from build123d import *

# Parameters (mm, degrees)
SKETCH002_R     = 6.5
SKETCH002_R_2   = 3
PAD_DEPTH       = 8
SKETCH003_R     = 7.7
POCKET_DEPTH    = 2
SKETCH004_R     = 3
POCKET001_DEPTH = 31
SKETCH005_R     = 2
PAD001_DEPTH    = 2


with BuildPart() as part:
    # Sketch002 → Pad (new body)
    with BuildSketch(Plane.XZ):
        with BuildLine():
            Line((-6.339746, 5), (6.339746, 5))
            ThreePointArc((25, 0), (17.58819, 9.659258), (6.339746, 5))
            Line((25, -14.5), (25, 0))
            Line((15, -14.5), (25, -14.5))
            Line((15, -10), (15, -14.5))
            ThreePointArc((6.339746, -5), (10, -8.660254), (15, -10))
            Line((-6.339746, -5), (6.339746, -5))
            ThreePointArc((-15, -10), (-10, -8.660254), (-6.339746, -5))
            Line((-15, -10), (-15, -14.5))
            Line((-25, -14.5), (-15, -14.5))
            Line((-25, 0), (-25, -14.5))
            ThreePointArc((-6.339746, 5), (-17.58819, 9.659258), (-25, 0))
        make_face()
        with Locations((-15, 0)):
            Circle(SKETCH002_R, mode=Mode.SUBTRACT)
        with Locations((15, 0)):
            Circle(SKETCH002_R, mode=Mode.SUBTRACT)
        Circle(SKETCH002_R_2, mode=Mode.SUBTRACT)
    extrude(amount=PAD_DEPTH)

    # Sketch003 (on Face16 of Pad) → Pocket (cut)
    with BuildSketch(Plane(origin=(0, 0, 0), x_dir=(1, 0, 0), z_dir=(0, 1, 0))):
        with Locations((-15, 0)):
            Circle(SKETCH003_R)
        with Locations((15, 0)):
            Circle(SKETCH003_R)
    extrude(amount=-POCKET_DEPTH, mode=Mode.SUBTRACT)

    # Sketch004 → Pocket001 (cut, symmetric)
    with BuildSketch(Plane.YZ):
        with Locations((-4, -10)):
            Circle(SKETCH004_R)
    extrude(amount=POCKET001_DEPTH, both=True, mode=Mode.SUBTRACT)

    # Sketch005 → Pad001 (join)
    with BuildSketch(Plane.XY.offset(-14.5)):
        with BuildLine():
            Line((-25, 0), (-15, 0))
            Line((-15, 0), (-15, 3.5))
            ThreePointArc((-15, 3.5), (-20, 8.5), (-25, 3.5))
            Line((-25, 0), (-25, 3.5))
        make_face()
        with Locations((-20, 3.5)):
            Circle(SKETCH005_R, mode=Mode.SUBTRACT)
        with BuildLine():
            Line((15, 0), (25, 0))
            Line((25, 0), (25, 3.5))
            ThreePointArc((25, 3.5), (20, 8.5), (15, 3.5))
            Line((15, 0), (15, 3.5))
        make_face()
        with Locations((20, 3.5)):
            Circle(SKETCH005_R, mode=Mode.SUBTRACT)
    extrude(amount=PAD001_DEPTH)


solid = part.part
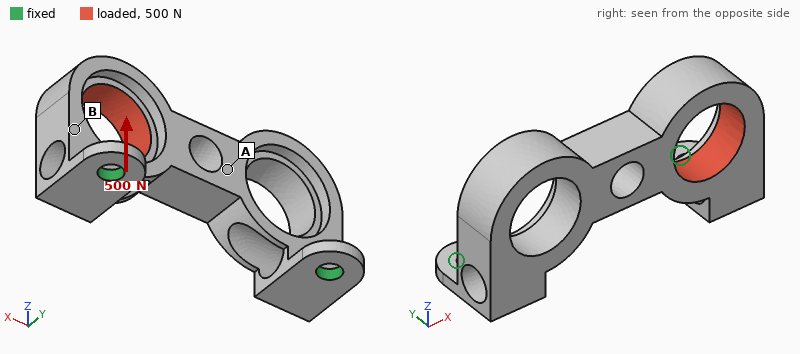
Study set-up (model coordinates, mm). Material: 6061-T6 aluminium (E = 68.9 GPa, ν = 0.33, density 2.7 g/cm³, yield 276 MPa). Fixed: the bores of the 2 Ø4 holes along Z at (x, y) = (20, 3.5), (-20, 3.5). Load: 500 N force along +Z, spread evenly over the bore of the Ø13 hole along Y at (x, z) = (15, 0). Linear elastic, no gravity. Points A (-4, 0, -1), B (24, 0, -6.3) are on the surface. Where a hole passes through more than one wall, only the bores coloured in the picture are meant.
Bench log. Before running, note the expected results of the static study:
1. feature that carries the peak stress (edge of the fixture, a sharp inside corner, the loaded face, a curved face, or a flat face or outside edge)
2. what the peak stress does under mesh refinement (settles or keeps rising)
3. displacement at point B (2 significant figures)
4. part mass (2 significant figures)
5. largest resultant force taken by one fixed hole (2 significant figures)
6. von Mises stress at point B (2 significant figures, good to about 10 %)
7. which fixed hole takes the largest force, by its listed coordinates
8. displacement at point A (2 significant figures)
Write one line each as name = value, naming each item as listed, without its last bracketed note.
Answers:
feature that carries the peak stress = a sharp inside corner
what the peak stress does under mesh refinement = keeps rising
displacement at point B = 0.099 mm
part mass = 11 g
largest resultant force taken by one fixed hole = 430 N
von Mises stress at point B = 46 MPa
which fixed hole takes the largest force, by its listed coordinates = (20, 3.5)
displacement at point A = 0.15 mm
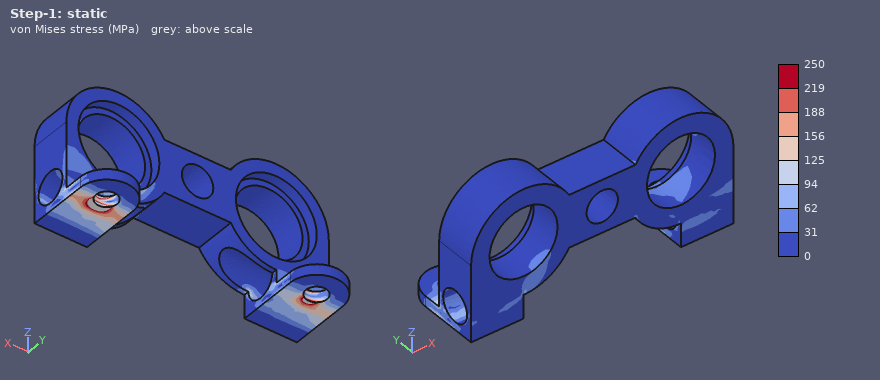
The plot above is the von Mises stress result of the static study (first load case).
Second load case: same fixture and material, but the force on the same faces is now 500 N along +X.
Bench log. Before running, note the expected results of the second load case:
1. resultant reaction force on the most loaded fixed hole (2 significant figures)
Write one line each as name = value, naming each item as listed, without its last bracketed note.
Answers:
resultant reaction force on the most loaded fixed hole = 300 N
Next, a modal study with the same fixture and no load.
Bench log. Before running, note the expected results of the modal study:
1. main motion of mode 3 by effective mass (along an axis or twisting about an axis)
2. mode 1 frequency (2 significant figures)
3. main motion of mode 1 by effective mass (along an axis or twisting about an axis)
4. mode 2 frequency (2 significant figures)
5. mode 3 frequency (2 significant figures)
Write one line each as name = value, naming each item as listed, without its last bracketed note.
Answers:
main motion of mode 3 by effective mass = along X
mode 1 frequency = 1600 Hz
main motion of mode 1 by effective mass = along Y
mode 2 frequency = 5200 Hz
mode 3 frequency = 8500 Hz
